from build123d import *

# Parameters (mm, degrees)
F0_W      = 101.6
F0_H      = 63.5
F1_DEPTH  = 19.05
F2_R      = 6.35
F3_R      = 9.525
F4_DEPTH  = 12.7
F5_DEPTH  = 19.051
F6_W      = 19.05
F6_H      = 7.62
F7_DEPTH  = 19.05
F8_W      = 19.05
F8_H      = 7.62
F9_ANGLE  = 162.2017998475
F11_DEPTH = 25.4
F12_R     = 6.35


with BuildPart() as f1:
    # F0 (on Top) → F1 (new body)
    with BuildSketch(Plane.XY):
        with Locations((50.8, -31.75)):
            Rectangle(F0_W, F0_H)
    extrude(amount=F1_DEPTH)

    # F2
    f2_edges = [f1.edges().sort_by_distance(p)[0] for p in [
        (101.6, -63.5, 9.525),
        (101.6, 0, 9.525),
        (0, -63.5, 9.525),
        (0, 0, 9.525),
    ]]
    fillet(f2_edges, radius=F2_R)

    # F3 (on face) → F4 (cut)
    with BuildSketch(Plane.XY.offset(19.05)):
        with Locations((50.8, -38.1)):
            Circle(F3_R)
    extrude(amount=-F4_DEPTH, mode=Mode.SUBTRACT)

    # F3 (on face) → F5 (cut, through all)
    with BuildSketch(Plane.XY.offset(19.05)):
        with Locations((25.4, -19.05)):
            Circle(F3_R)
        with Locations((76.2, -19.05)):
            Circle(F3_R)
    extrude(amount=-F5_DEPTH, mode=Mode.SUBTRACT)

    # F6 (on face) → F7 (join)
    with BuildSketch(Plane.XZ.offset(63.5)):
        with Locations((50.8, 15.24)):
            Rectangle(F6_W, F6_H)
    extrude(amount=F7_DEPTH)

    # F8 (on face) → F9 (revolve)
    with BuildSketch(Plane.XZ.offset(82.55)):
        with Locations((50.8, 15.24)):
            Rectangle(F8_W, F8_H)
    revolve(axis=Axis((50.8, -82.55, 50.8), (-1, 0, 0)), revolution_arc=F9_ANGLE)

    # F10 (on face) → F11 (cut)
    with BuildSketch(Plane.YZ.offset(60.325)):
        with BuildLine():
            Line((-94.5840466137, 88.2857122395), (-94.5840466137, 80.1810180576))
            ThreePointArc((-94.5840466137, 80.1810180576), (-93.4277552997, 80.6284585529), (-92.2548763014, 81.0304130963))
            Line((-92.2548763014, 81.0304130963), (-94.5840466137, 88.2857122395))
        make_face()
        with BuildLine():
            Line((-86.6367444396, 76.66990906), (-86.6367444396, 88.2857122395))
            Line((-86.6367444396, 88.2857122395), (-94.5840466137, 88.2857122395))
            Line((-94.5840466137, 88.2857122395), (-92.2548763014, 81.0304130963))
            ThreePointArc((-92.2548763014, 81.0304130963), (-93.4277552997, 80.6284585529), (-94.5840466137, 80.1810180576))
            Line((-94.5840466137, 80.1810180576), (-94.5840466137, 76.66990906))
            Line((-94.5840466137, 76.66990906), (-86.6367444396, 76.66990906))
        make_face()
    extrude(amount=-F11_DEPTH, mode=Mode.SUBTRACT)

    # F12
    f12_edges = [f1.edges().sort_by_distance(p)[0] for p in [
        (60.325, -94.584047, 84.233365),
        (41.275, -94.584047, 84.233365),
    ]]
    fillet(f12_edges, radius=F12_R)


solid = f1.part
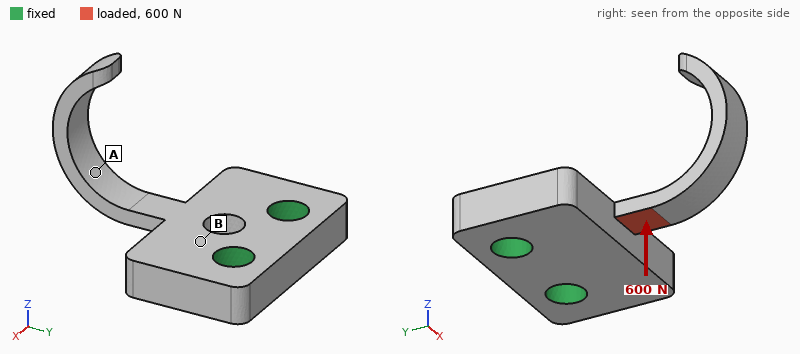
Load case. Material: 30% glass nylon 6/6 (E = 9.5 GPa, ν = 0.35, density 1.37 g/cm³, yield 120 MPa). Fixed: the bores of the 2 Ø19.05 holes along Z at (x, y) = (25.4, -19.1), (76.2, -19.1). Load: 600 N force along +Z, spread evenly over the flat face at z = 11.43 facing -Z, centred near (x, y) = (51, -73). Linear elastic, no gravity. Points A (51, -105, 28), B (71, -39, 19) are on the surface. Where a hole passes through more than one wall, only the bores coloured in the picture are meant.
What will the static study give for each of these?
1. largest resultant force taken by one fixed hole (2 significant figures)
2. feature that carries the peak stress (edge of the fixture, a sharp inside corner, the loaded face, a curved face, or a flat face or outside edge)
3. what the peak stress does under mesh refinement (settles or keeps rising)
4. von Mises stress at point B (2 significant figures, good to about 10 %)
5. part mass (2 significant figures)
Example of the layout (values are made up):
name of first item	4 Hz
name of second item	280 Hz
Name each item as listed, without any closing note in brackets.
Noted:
largest resultant force taken by one fixed hole	300 N
feature that carries the peak stress	a sharp inside corner
what the peak stress does under mesh refinement	keeps rising
von Mises stress at point B	5.1 MPa
part mass	170 g
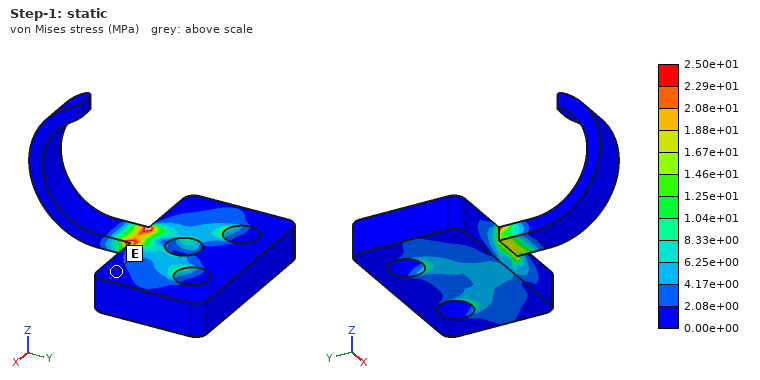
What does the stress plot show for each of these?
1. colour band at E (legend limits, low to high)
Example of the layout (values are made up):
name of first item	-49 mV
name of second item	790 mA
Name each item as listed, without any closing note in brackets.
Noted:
colour band at E	0.00e+00 to 2.08e+00 MPa
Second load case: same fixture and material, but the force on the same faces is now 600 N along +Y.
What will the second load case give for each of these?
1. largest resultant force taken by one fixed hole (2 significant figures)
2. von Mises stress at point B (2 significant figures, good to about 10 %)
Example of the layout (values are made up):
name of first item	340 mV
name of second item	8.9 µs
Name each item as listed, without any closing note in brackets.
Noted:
largest resultant force taken by one fixed hole	330 N
von Mises stress at point B	1.1 MPa
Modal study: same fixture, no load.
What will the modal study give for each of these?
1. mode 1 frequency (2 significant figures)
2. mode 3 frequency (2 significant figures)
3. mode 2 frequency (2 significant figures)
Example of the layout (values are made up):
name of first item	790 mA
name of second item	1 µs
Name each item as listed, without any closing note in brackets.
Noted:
mode 1 frequency	270 Hz
mode 3 frequency	800 Hz
mode 2 frequency	380 Hz
